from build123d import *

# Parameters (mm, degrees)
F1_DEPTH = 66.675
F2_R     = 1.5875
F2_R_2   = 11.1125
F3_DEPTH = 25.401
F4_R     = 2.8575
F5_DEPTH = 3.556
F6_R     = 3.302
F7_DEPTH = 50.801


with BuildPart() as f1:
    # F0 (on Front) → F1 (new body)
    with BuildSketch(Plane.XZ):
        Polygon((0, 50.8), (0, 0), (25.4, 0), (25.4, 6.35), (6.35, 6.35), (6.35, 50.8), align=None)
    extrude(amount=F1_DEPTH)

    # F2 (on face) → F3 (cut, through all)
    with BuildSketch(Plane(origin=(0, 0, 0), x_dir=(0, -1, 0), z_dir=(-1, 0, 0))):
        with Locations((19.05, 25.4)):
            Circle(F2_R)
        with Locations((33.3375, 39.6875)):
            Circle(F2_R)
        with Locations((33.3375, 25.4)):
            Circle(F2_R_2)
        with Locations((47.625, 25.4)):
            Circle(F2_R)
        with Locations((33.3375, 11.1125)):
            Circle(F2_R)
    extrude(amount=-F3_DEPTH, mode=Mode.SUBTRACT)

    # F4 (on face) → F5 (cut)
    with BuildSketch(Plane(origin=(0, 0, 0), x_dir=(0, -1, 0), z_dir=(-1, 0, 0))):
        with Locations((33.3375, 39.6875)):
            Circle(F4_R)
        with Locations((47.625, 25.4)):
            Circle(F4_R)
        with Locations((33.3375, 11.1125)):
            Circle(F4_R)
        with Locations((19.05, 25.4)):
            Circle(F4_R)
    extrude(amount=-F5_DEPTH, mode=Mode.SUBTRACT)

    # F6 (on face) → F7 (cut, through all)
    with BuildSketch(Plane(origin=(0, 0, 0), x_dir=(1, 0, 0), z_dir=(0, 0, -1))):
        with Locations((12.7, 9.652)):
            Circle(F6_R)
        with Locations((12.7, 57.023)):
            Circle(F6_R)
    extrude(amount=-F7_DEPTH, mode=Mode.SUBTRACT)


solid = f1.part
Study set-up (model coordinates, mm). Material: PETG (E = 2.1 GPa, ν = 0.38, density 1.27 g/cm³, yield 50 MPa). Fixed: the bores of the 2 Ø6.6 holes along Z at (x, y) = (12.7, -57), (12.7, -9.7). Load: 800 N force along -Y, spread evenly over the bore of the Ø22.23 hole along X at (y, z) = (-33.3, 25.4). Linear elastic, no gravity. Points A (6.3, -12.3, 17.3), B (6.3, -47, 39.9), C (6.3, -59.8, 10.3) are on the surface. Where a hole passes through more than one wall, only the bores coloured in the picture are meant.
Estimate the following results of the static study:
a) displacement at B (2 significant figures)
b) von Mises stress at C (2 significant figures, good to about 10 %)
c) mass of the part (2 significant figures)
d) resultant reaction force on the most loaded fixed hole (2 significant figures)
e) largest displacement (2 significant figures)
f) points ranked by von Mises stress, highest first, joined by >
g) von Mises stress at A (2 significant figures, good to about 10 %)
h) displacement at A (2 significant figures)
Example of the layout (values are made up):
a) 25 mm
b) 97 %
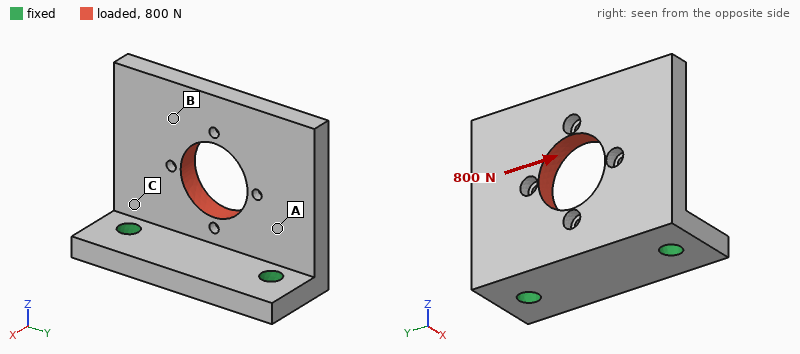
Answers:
a) 0.32 mm
b) 7.1 MPa
c) 33 g
d) 540 N
e) 0.44 mm
f) C > A > B
g) 5.3 MPa
h) 0.16 mm
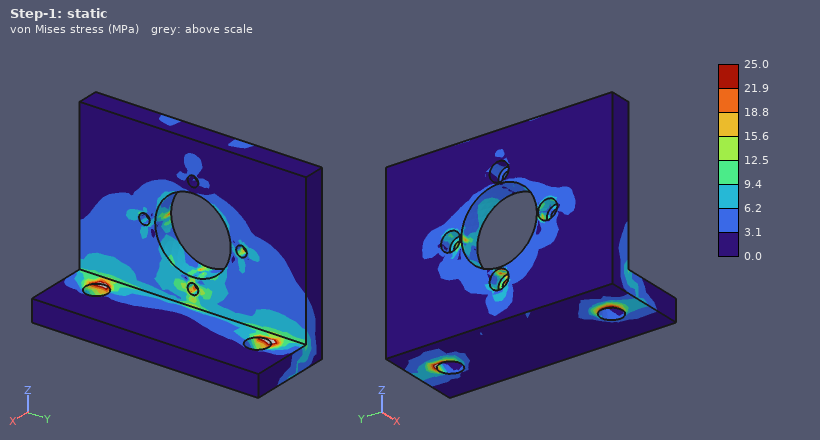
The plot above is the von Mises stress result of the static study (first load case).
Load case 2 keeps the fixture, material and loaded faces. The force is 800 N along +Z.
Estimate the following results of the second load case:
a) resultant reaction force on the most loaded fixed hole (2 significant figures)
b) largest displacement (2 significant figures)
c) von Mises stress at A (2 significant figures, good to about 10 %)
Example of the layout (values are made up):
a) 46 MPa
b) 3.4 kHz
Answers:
a) 410 N
b) 0.72 mm
c) 2.8 MPa
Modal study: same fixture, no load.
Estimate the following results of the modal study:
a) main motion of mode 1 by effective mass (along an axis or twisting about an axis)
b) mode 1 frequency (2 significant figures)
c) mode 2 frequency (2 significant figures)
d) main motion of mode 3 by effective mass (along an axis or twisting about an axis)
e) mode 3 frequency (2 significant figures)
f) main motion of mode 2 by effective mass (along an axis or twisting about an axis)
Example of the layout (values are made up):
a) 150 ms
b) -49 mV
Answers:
a) along X
b) 440 Hz
c) 870 Hz
d) along Y
e) 1700 Hz
f) twisting about Z
